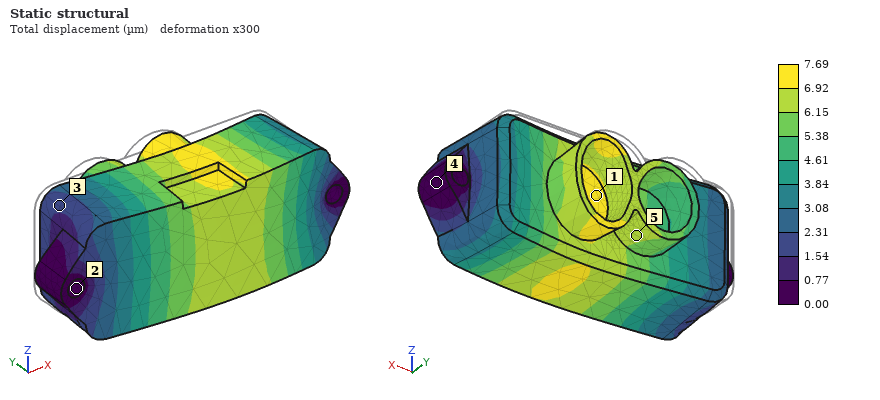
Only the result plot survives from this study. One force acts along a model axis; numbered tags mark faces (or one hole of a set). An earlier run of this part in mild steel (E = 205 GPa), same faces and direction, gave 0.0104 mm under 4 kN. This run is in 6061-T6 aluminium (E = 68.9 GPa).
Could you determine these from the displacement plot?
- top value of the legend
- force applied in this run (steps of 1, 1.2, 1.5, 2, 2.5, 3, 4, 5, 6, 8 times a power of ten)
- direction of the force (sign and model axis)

7.69 µm
1 kN
-Y
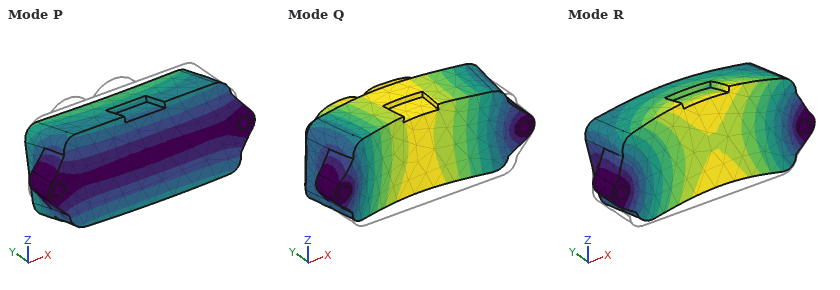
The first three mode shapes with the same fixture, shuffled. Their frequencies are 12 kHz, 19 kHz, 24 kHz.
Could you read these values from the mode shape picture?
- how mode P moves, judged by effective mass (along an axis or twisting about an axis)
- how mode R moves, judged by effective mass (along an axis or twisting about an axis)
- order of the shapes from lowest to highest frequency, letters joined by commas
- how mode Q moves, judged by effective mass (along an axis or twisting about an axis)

along Z
along Z
P, Q, R
along Y
